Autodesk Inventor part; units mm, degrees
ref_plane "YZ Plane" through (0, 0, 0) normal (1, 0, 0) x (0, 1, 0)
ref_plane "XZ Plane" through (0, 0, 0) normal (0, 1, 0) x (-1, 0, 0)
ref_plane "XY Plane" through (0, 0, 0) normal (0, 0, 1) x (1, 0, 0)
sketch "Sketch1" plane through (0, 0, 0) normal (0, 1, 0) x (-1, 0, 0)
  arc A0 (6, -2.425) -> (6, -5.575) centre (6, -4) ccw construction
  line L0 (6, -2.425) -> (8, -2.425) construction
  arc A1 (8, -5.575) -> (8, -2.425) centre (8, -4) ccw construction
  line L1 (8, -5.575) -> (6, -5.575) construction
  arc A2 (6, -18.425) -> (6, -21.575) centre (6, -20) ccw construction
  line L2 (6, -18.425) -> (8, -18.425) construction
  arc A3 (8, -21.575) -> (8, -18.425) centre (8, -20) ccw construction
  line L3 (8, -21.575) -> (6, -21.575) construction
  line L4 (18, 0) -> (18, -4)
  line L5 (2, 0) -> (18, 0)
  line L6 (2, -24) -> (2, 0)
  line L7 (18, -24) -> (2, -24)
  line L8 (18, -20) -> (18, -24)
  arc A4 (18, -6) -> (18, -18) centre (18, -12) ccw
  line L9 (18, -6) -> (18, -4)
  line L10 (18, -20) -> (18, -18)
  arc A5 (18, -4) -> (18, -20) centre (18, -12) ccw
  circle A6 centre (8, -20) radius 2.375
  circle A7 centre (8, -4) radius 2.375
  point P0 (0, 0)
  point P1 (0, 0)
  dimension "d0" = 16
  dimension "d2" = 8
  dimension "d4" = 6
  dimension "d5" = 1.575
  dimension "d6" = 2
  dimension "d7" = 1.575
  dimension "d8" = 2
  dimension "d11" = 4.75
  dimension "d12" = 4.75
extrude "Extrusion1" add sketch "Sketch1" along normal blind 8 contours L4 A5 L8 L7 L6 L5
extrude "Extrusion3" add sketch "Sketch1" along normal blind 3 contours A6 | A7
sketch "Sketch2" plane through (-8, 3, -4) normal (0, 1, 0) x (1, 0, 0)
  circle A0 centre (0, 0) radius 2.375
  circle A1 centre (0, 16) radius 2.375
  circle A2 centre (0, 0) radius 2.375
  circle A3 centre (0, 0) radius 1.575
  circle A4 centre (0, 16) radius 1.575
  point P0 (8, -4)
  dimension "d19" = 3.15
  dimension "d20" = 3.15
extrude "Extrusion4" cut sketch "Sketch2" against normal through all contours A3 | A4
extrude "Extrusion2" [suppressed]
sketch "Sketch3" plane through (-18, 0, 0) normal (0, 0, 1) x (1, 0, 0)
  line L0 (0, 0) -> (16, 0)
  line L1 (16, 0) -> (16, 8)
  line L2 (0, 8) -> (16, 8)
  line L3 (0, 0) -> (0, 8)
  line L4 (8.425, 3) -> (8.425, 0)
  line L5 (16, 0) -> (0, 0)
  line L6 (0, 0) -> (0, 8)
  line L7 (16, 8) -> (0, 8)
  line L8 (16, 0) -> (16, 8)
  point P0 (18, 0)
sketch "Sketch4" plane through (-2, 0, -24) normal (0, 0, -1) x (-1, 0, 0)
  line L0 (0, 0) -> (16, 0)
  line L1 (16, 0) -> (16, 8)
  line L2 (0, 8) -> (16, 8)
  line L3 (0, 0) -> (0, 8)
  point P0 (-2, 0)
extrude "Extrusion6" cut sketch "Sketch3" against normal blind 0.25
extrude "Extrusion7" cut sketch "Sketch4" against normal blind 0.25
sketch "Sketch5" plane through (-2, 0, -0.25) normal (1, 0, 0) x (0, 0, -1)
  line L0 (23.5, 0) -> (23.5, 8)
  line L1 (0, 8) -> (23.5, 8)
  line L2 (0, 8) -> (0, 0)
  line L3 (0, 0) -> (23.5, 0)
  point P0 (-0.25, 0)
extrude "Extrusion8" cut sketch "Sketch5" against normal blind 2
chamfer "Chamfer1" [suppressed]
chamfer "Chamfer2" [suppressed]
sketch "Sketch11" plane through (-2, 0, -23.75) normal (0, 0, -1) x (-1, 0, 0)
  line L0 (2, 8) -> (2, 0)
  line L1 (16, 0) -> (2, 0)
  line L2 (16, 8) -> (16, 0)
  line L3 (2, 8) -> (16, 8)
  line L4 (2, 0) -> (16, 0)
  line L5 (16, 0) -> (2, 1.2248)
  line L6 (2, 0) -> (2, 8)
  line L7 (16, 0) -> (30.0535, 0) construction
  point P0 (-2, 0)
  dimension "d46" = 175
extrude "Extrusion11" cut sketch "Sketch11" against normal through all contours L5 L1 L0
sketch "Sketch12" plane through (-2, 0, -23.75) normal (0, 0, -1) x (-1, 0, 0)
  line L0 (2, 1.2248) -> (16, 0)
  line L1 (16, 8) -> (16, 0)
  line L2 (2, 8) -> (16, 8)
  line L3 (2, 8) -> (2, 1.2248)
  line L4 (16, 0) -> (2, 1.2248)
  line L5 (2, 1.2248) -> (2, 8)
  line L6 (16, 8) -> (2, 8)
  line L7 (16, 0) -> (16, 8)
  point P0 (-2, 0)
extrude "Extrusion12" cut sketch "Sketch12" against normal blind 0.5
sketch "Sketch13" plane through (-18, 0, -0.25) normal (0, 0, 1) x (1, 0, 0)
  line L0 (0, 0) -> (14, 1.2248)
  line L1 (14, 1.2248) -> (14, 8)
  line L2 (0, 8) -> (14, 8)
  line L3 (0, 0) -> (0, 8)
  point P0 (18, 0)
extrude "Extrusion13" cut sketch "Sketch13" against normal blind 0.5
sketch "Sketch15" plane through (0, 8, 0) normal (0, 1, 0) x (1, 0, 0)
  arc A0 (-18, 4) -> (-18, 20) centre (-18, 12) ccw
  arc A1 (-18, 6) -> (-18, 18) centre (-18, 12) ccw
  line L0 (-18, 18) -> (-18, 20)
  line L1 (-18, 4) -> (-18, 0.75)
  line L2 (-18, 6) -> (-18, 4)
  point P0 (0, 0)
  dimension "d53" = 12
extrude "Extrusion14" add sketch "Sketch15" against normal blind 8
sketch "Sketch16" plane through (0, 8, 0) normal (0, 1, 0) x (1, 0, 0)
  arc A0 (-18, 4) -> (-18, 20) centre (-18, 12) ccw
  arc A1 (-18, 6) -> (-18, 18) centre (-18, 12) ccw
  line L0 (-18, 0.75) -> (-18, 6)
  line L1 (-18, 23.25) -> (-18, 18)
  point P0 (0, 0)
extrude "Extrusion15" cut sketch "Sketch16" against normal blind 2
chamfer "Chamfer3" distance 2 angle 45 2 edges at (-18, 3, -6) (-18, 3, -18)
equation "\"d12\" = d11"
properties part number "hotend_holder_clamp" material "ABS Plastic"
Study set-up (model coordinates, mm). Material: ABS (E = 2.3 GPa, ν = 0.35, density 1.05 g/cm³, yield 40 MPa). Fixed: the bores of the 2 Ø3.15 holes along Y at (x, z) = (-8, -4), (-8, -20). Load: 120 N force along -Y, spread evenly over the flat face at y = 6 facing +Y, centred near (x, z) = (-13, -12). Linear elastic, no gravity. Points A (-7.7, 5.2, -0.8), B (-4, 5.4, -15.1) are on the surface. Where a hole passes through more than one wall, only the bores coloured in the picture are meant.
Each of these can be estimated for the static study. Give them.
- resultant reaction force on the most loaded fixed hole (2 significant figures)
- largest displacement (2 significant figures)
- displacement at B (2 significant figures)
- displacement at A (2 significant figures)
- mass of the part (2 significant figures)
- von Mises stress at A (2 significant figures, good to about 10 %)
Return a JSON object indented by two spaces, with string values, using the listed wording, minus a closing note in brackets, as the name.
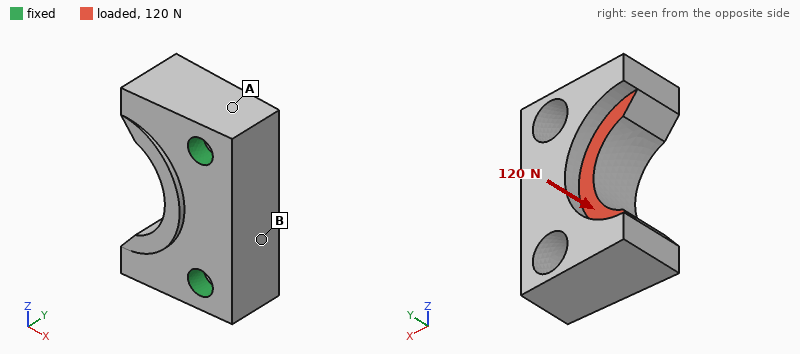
{
  "resultant reaction force on the most loaded fixed hole": "64 N",
  "largest displacement": "0.12 mm",
  "displacement at B": "0.039 mm",
  "displacement at A": "0.029 mm",
  "mass of the part": "1.7 g",
  "von Mises stress at A": "6.3 MPa"
}
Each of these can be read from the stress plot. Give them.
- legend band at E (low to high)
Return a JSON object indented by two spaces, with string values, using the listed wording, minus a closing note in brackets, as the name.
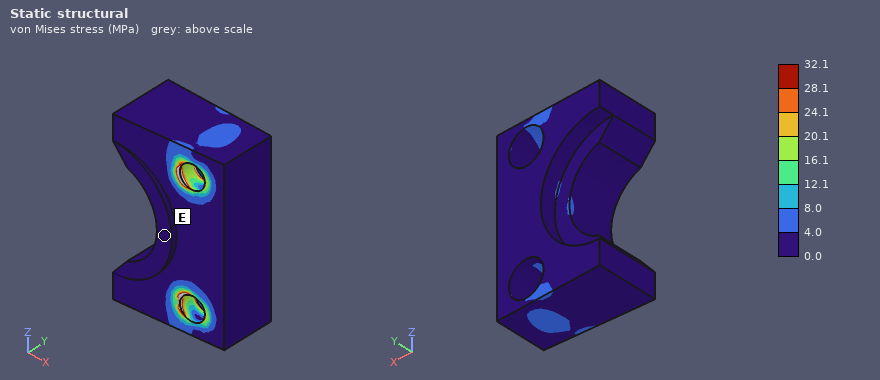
{
  "legend band at E": "0.0 to 4.0 MPa"
}
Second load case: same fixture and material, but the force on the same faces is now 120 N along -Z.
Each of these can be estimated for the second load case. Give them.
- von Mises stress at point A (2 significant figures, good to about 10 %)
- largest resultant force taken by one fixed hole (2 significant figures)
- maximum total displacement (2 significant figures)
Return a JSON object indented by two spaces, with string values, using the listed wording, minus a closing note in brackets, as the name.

{
  "von Mises stress at point A": "1.5 MPa",
  "largest resultant force taken by one fixed hole": "73 N",
  "maximum total displacement": "30 µm"
}
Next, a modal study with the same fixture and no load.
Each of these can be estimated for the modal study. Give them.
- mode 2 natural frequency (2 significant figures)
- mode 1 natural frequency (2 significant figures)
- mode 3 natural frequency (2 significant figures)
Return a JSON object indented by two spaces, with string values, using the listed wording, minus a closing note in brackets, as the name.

{
  "mode 2 natural frequency": "9200 Hz",
  "mode 1 natural frequency": "5900 Hz",
  "mode 3 natural frequency": "12 kHz"
}
